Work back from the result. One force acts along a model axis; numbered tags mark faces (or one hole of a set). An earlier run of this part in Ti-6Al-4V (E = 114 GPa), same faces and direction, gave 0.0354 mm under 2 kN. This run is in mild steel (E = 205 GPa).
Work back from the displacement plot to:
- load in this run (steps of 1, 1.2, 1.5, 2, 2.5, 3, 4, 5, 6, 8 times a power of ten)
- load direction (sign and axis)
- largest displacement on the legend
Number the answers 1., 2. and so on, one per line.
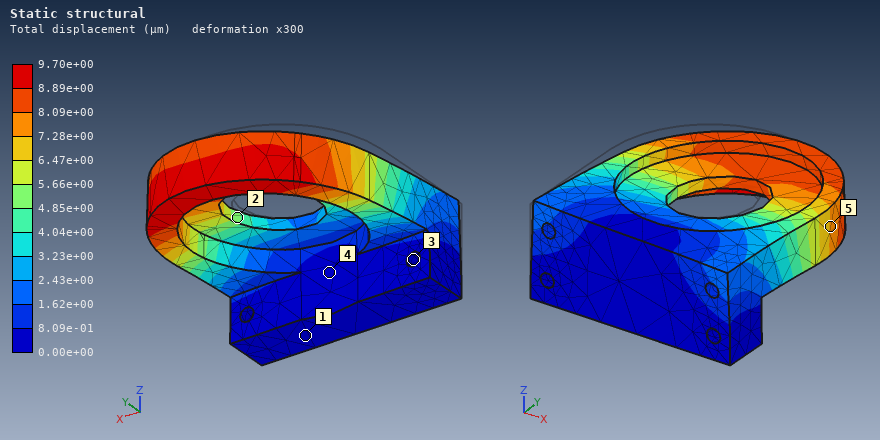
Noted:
1. 1 kN
2. +X
3. 9.70e+00 µm
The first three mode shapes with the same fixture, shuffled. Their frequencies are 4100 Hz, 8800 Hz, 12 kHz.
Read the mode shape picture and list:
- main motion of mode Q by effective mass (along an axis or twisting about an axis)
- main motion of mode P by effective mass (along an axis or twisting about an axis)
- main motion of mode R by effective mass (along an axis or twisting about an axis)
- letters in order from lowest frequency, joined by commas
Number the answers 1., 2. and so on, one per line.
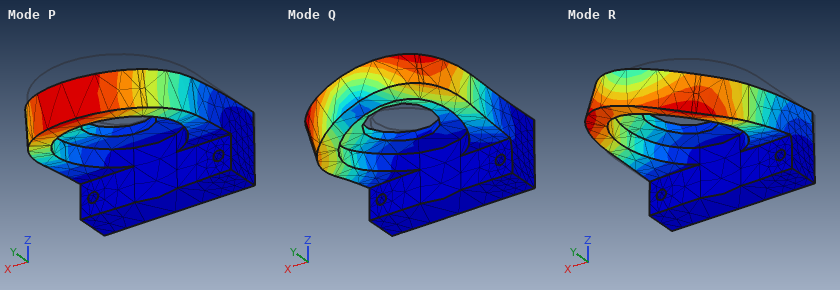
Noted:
1. along X
2. along Z
3. along X
4. P, R, Q
